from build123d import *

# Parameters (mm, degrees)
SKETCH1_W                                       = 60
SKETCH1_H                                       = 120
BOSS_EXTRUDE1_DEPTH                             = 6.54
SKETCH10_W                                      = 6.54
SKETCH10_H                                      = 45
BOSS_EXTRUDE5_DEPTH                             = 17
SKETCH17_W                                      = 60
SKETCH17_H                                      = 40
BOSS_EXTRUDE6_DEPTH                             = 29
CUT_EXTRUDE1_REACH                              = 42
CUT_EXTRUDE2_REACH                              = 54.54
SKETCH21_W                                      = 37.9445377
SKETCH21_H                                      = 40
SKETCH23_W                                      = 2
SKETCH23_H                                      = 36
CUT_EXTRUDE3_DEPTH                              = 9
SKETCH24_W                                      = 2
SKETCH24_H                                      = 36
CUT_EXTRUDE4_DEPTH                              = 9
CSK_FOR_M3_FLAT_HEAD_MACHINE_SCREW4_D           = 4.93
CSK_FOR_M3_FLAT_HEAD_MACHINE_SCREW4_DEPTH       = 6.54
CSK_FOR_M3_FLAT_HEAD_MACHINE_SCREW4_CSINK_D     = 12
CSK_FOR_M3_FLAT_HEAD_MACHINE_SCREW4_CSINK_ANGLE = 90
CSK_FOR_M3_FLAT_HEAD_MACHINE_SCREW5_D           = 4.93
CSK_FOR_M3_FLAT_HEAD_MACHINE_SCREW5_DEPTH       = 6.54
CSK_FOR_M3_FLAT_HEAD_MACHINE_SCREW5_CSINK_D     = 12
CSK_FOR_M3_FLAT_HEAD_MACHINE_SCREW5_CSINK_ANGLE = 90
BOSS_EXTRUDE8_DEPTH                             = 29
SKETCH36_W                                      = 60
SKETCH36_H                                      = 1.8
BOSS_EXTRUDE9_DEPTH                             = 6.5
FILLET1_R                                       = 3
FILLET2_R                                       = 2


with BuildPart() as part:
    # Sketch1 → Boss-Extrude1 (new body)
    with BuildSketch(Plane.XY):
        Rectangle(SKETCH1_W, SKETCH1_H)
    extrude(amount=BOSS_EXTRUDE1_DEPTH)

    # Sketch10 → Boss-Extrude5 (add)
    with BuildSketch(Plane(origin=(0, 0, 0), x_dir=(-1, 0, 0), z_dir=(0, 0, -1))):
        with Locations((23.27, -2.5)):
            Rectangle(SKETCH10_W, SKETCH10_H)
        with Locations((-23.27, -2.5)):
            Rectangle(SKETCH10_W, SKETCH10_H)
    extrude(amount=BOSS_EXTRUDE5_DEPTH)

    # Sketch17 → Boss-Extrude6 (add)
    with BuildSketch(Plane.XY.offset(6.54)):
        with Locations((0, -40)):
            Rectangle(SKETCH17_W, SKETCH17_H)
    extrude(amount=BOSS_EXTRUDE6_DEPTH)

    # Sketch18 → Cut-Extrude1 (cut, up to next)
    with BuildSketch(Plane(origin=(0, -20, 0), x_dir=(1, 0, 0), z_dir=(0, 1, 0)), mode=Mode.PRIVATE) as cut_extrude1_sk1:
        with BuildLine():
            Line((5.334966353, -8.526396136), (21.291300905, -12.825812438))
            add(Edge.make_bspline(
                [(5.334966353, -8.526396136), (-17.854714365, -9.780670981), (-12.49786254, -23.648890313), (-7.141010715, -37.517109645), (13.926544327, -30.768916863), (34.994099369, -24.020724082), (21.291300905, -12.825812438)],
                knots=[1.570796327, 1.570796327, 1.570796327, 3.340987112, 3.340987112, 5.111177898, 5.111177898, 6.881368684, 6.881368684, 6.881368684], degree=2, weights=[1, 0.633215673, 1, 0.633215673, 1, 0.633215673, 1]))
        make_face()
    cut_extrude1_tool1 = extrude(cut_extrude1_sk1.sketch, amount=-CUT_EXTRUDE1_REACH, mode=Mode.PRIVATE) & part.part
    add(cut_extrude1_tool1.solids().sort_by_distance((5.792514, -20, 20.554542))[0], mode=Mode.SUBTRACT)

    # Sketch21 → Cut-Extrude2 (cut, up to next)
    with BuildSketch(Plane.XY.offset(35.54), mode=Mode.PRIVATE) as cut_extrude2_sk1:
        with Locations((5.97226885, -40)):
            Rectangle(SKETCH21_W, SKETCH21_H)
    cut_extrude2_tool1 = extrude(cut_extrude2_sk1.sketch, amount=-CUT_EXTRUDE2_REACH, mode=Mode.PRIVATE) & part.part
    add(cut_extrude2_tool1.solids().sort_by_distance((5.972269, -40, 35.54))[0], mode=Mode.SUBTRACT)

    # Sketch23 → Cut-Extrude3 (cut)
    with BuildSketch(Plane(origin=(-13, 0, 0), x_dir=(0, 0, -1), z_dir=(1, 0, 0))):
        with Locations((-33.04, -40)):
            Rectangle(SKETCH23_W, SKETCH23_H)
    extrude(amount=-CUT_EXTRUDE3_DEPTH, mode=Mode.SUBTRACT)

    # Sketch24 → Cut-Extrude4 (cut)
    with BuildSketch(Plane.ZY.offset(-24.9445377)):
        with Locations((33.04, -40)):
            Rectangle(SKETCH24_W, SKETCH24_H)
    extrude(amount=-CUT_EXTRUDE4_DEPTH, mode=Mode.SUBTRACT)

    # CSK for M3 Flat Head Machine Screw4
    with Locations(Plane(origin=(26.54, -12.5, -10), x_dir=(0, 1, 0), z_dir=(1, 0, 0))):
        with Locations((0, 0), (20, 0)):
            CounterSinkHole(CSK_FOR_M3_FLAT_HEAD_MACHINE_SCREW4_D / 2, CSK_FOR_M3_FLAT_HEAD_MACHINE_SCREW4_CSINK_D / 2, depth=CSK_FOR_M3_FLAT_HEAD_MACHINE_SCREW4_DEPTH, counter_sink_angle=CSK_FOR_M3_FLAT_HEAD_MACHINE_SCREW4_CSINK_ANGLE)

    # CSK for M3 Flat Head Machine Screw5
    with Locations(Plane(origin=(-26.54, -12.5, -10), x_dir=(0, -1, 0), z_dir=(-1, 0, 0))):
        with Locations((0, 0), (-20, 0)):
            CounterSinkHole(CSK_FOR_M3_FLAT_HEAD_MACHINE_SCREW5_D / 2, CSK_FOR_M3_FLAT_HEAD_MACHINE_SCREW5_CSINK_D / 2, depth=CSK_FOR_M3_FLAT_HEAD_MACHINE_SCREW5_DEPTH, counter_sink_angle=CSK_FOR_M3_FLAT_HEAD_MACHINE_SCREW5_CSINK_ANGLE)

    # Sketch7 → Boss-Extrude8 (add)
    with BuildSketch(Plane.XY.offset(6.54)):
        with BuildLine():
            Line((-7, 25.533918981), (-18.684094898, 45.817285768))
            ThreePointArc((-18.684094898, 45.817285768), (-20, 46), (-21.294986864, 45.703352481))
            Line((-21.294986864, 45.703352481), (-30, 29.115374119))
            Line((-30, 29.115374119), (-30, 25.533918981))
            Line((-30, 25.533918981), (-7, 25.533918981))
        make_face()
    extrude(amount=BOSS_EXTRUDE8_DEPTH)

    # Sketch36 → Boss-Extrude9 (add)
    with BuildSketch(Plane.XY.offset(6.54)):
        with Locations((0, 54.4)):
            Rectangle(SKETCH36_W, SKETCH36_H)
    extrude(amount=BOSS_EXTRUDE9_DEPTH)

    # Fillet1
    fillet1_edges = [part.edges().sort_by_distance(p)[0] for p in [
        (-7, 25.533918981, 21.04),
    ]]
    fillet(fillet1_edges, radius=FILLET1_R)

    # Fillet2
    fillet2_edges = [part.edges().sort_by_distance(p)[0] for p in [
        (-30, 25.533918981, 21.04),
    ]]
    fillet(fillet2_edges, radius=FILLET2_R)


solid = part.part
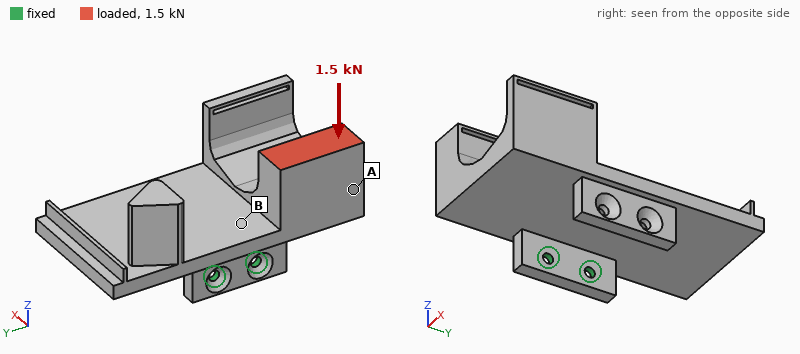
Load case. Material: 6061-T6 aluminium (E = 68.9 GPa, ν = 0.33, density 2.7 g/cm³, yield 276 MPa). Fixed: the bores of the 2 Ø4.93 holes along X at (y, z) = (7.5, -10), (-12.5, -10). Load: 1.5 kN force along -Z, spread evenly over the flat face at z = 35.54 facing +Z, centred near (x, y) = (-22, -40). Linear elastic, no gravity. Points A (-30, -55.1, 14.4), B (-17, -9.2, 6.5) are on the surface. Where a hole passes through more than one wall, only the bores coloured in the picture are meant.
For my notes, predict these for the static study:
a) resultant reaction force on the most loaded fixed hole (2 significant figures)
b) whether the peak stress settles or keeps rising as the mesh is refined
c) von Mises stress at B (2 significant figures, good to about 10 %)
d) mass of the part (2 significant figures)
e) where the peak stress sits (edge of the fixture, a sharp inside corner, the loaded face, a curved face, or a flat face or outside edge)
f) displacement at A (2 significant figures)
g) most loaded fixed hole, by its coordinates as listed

3.2 kN
keeps rising
32 MPa
260 g
edge of the fixture
0.14 mm
(-12.5, -10)
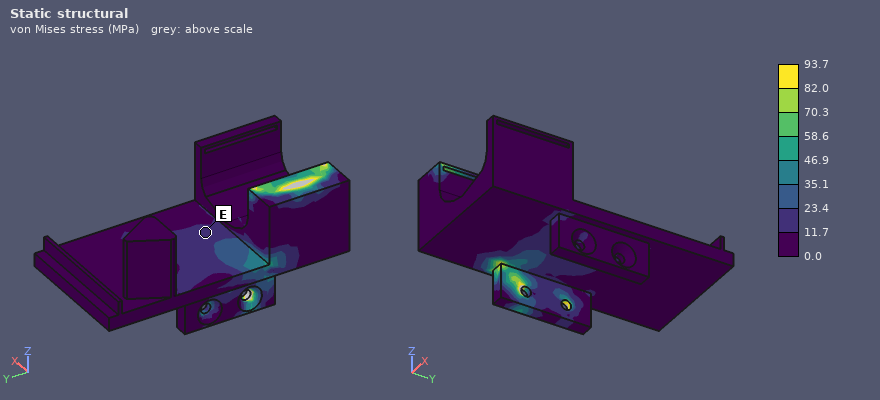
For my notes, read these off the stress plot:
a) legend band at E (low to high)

11.7 to 23.4 MPa
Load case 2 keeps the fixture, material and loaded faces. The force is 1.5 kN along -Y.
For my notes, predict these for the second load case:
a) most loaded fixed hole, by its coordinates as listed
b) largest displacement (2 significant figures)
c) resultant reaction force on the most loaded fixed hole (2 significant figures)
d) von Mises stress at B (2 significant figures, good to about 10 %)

(7.5, -10)
0.33 mm
3.2 kN
48 MPa
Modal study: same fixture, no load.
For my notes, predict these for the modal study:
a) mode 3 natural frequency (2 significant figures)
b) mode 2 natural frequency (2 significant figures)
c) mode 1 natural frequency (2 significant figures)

1100 Hz
880 Hz
510 Hz
